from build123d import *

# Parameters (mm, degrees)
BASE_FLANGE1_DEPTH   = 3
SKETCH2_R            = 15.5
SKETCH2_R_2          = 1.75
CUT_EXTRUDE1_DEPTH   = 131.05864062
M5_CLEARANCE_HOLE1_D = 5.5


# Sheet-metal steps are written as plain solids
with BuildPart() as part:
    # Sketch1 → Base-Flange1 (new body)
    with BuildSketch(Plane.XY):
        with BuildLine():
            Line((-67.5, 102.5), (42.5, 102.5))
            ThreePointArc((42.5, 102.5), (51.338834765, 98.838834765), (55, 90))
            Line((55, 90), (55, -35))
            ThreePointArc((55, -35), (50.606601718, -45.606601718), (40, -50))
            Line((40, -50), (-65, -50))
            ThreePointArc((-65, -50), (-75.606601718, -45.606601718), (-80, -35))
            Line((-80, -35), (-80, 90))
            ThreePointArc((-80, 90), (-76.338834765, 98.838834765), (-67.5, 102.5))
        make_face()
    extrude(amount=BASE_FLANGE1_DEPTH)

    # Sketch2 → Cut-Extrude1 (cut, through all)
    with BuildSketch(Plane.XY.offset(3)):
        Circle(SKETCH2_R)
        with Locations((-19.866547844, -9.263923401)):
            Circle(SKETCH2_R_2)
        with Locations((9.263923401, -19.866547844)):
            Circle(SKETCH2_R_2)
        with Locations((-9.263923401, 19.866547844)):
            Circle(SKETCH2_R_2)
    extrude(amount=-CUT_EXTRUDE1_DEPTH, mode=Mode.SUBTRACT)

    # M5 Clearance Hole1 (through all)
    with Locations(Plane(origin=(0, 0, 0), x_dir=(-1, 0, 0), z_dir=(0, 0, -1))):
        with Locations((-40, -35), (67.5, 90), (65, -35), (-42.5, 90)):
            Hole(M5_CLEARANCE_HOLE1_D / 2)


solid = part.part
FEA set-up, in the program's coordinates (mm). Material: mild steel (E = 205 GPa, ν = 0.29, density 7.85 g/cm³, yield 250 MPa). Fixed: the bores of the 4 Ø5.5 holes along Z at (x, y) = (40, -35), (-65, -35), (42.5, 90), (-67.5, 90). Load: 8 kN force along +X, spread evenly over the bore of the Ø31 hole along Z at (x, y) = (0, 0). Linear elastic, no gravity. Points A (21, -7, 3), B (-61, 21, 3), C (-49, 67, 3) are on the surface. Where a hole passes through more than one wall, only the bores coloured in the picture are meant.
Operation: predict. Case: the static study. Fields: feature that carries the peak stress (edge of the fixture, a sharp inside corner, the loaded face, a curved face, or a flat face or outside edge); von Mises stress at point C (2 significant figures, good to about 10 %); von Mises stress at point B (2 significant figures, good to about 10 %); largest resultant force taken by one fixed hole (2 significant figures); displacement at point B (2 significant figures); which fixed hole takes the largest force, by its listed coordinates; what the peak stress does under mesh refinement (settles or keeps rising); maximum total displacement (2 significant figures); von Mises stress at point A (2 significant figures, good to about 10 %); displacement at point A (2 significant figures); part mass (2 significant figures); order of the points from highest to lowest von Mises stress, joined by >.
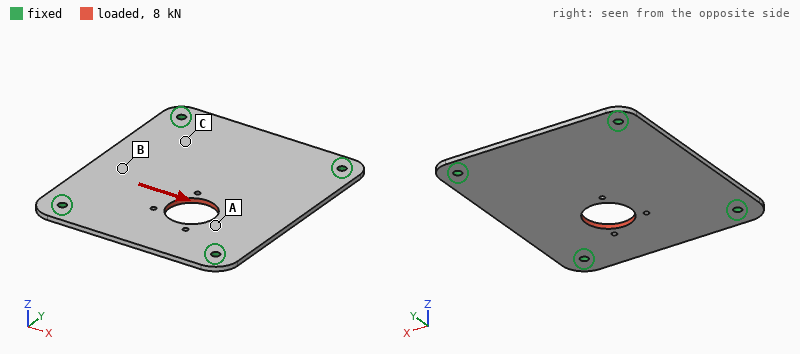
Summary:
edge of the fixture
16 MPa
6.7 MPa
3.0 kN
7.3 µm
(40, -35)
keeps rising
13 µm
28 MPa
9.7 µm
460 g
A > C > B
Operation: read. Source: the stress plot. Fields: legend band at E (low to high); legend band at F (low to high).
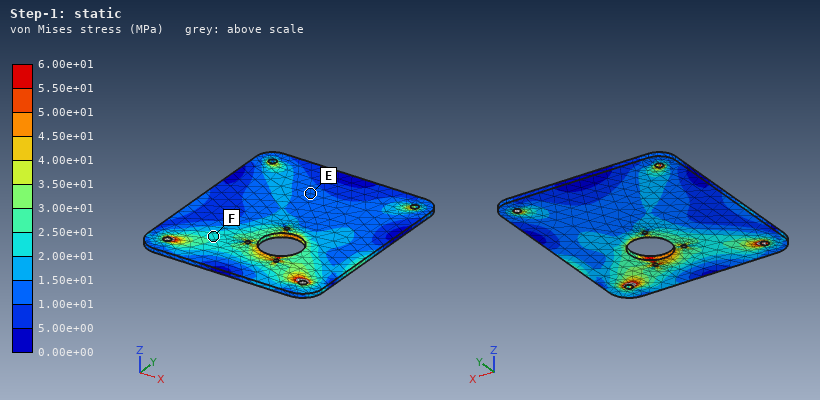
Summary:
1.00e+01 to 1.50e+01 MPa
2.00e+01 to 2.50e+01 MPa
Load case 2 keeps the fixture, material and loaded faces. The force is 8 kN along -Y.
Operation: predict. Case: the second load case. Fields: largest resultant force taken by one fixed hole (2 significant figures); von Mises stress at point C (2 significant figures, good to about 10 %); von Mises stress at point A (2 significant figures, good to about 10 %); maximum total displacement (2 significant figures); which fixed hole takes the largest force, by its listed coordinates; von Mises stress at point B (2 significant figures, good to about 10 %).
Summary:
2.9 kN
15 MPa
33 MPa
13 µm
(40, -35)
8.8 MPa
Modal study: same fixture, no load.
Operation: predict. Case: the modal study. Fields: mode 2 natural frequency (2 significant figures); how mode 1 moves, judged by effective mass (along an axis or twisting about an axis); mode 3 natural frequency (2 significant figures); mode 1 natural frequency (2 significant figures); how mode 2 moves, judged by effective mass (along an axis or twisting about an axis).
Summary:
1200 Hz
along Z
1400 Hz
760 Hz
twisting about Y
